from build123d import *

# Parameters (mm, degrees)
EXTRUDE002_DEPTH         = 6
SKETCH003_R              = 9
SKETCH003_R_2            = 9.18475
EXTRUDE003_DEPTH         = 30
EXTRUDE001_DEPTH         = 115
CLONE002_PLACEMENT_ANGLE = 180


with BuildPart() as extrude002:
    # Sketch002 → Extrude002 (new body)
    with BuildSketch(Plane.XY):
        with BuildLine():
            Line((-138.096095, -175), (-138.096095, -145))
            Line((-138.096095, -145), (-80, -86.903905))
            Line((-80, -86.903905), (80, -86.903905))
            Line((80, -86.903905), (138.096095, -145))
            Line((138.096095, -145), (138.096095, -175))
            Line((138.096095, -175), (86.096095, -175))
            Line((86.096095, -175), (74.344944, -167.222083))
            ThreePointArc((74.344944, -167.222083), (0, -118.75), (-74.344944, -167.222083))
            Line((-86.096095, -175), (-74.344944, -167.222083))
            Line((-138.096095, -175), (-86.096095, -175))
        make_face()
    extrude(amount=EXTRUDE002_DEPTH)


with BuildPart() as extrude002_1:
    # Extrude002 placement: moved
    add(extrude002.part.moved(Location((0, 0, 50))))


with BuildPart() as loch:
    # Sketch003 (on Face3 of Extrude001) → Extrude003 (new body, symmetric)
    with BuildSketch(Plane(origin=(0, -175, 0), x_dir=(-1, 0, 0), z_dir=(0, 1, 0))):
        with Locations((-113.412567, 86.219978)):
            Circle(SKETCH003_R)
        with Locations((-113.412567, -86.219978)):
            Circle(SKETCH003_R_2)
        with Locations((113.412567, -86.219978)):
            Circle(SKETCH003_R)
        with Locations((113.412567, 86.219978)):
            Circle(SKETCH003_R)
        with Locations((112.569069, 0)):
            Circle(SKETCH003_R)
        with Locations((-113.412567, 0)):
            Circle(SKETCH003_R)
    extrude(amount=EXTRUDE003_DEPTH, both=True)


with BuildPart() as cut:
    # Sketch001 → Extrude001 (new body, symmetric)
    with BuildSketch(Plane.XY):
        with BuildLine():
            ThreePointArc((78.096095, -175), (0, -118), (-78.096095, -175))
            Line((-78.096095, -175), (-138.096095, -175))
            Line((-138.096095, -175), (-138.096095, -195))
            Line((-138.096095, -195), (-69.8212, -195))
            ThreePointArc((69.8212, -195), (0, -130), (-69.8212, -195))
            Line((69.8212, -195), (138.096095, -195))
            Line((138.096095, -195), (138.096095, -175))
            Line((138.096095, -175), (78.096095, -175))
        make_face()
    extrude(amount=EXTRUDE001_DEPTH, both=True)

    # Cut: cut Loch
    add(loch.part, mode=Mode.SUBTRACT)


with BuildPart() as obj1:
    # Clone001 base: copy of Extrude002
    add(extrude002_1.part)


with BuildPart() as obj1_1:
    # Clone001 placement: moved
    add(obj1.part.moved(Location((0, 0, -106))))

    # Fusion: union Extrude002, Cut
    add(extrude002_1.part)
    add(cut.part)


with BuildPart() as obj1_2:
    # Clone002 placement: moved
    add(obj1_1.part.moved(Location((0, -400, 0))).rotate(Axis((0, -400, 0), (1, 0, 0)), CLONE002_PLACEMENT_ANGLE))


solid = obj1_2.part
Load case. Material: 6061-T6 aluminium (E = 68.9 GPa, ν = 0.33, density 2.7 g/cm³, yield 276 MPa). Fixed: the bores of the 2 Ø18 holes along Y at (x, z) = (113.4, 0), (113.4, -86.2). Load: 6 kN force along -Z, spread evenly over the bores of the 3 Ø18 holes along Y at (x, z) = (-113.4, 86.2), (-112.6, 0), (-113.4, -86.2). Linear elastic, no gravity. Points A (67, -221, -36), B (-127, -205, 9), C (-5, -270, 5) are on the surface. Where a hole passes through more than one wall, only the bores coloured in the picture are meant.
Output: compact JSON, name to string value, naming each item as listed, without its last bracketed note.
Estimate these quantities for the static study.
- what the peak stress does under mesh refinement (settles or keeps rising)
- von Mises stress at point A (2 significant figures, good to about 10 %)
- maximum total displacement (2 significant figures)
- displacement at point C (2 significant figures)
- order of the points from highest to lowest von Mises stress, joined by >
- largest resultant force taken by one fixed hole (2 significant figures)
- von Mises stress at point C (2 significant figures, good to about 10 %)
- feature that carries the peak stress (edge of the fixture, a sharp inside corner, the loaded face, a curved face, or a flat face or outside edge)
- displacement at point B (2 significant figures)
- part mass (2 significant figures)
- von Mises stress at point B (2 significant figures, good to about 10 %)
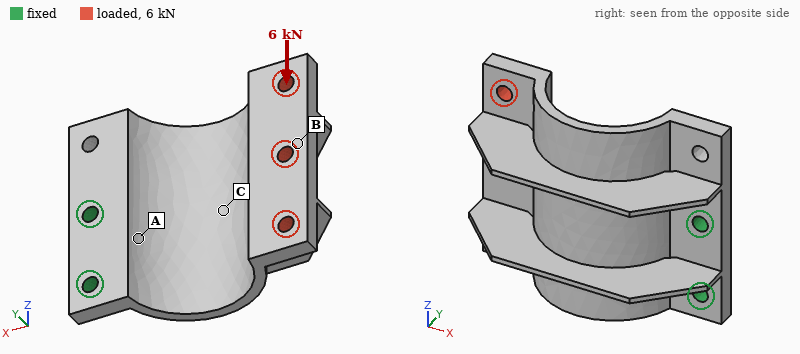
{"what the peak stress does under mesh refinement": "keeps rising", "von Mises stress at point A": "44 MPa", "maximum total displacement": "1.7 mm", "displacement at point C": "0.28 mm", "order of the points from highest to lowest von Mises stress, joined by >": "A > C > B", "largest resultant force taken by one fixed hole": "14 kN", "von Mises stress at point C": "29 MPa", "feature that carries the peak stress": "edge of the fixture", "displacement at point B": "1.2 mm", "part mass": "3.5 kg", "von Mises stress at point B": "11 MPa"}
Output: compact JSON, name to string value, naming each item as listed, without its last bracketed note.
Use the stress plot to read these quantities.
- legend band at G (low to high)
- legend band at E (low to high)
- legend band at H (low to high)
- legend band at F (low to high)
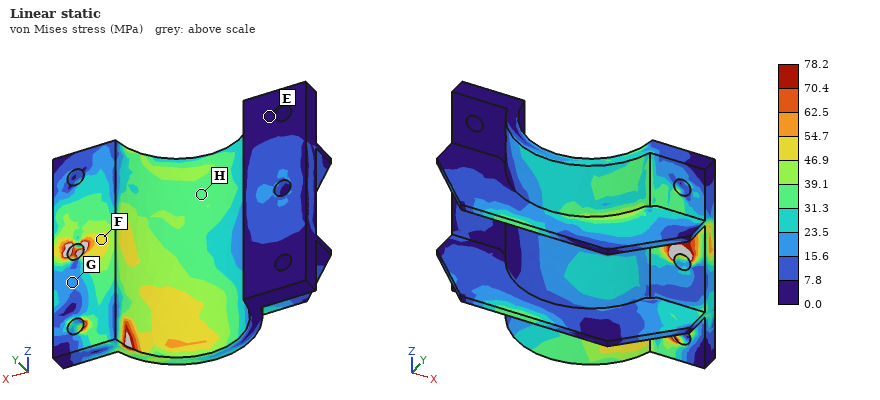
{"legend band at G": "15.6 to 23.5 MPa", "legend band at E": "0.0 to 7.8 MPa", "legend band at H": "31.3 to 39.1 MPa", "legend band at F": "46.9 to 54.7 MPa"}
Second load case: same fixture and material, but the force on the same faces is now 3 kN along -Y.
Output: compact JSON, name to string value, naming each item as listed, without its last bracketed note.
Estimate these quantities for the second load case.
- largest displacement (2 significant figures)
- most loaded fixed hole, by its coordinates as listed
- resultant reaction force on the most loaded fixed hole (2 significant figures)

{"largest displacement": "1.3 mm", "most loaded fixed hole, by its coordinates as listed": "(113.4, 0)", "resultant reaction force on the most loaded fixed hole": "3.7 kN"}
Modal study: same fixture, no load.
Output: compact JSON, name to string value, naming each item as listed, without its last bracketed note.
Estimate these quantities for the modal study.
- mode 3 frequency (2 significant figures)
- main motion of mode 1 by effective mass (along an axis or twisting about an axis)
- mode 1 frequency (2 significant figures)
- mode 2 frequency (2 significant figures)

{"mode 3 frequency": "660 Hz", "main motion of mode 1 by effective mass": "along Y", "mode 1 frequency": "240 Hz", "mode 2 frequency": "330 Hz"}
